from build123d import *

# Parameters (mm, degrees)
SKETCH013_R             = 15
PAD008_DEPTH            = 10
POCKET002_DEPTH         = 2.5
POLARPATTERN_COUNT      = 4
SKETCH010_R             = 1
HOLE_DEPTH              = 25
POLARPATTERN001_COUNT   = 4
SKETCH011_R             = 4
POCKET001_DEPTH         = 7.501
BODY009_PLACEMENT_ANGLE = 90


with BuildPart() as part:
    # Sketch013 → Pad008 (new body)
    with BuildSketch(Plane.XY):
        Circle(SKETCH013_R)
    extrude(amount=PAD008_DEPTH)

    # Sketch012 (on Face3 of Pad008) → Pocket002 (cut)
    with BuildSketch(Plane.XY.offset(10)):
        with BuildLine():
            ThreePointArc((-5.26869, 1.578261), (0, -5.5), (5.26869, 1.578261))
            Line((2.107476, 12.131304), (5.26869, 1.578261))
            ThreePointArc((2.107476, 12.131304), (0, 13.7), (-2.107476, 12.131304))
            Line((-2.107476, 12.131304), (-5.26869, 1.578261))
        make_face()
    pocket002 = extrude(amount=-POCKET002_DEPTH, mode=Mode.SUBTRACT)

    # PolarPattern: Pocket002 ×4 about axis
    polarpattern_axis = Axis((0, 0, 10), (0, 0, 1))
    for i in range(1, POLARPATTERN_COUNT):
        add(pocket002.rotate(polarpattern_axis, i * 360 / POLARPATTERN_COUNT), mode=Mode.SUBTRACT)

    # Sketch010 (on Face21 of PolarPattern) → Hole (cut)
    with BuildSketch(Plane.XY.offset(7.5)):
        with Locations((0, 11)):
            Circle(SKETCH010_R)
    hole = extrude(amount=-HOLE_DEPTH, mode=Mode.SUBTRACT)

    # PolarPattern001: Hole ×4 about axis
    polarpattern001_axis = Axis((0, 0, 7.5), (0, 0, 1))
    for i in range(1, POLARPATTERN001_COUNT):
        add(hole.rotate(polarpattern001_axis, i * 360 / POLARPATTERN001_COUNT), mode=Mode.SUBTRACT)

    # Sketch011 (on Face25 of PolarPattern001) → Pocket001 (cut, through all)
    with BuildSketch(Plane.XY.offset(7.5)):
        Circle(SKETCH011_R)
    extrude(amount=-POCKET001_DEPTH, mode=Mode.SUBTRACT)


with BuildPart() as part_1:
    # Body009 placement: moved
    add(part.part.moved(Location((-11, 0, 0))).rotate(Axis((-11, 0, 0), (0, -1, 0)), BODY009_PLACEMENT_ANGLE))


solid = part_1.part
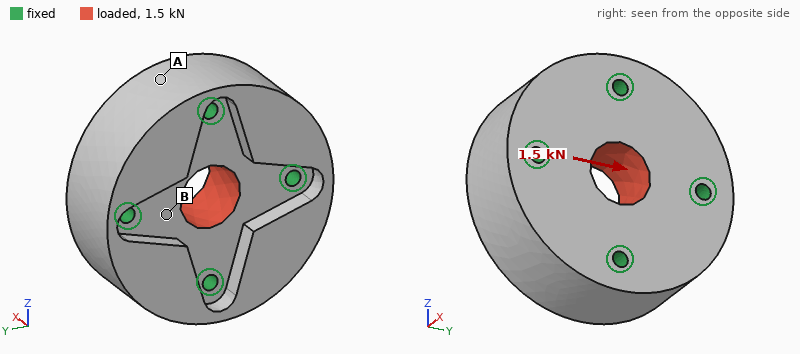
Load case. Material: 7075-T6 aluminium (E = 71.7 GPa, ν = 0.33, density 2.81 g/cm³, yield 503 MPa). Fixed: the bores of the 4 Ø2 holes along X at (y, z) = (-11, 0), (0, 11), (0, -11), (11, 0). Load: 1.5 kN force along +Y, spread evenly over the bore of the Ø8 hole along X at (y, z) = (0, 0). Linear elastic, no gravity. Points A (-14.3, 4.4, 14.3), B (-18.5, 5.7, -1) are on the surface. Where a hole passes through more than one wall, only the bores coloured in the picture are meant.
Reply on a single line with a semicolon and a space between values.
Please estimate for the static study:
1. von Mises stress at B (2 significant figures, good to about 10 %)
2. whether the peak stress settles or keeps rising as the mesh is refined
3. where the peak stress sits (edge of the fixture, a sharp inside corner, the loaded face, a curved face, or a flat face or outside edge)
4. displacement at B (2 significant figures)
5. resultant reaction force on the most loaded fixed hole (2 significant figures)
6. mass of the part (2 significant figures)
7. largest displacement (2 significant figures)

9.7 MPa; keeps rising; edge of the fixture; 0.70 µm; 460 N; 16 g; 1.1 µm
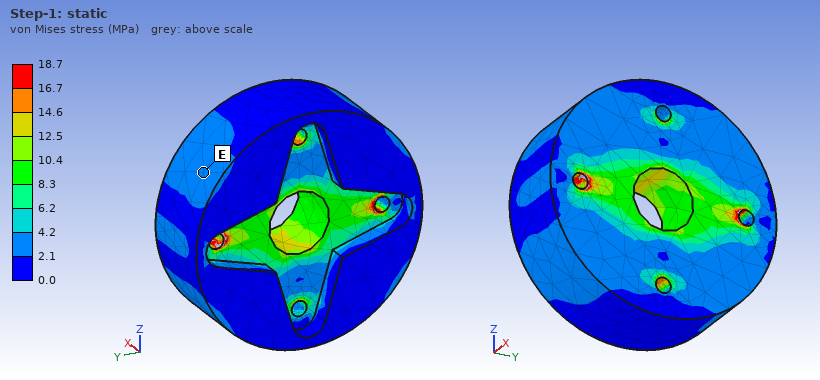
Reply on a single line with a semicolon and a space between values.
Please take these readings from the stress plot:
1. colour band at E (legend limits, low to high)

2.1 to 4.2 MPa
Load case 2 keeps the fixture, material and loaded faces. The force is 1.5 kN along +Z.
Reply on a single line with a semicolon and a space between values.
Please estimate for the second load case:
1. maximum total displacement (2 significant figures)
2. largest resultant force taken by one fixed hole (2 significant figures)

1.1 µm; 460 N
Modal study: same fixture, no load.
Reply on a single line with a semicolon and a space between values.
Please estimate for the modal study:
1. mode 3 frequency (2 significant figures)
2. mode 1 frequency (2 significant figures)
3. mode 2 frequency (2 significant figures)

52 kHz; 49 kHz; 52 kHz
